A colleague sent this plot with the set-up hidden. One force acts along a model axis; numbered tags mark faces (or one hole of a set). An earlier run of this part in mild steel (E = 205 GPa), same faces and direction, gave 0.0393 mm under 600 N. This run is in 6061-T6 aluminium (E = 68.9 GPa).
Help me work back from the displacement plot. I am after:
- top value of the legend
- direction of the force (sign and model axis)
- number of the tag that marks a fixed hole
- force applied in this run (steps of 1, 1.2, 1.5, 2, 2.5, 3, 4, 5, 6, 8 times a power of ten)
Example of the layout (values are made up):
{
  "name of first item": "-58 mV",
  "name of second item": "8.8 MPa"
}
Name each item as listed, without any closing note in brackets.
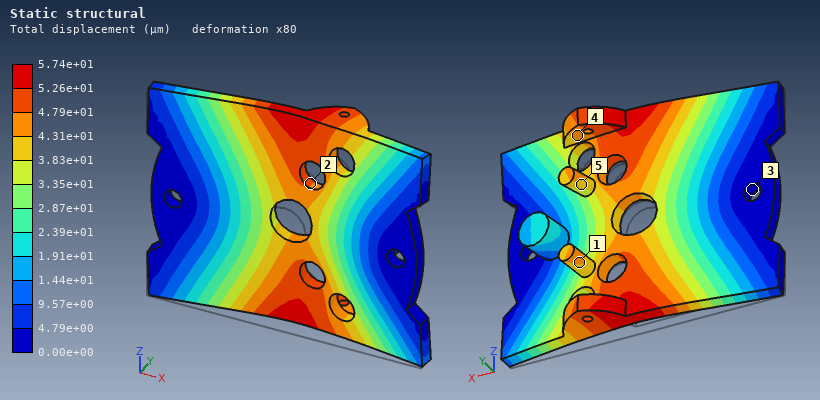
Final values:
{
  "top value of the legend": "5.74e+01 µm",
  "direction of the force": "+Y",
  "number of the tag that marks a fixed hole": "3",
  "force applied in this run": "300 N"
}
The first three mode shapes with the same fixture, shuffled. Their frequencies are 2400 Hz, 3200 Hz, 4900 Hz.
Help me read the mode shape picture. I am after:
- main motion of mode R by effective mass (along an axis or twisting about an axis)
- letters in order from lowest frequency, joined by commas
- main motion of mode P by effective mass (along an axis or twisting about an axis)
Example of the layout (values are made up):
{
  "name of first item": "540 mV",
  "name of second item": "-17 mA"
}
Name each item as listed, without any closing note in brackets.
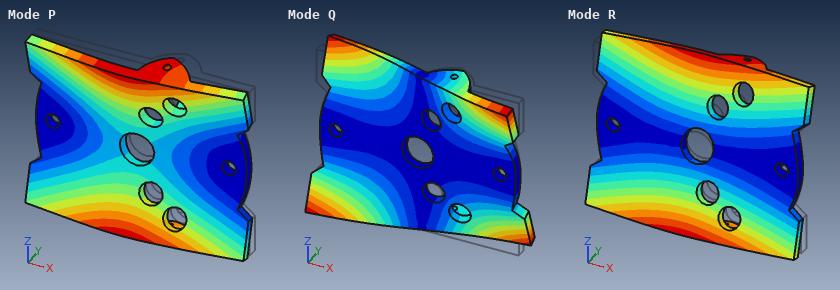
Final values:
{
  "main motion of mode R by effective mass": "twisting about X",
  "letters in order from lowest frequency, joined by commas": "R, P, Q",
  "main motion of mode P by effective mass": "along Y"
}
